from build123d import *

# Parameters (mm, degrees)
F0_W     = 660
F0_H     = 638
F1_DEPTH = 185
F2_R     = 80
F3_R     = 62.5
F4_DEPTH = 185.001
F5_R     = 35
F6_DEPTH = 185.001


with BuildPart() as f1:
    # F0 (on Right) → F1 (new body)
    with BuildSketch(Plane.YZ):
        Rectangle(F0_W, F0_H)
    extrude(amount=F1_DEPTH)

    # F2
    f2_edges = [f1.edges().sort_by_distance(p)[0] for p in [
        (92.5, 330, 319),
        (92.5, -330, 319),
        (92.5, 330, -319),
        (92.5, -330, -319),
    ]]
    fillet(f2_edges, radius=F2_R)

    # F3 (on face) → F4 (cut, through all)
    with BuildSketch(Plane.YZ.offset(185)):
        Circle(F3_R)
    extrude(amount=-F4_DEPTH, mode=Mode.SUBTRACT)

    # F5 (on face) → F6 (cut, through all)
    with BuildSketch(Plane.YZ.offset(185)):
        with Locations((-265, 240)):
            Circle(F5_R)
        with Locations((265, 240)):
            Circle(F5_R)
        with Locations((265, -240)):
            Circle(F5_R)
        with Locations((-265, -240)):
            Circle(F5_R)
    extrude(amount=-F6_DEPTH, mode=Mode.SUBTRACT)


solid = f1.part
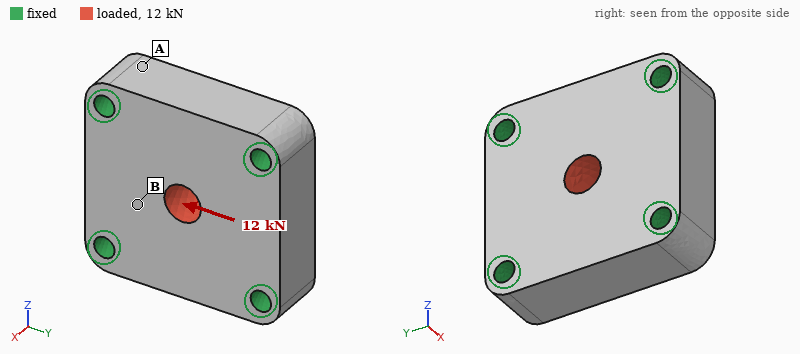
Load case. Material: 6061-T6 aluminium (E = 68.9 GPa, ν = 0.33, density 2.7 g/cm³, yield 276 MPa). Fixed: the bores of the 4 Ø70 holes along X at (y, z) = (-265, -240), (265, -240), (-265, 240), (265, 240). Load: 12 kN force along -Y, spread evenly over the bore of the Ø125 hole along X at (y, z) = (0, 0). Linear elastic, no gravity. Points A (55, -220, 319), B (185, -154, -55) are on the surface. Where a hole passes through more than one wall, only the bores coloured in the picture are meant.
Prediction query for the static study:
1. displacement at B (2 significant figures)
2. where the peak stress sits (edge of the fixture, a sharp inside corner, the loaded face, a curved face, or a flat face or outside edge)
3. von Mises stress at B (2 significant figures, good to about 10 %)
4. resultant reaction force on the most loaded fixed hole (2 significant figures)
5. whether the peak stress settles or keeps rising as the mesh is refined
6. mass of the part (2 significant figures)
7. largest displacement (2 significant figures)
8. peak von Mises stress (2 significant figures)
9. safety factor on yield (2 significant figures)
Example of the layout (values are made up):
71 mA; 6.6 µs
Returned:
0.42 µm; the loaded face; 0.096 MPa; 3.3 kN; settles; 190 kg; 0.63 µm; 0.29 MPa; 950
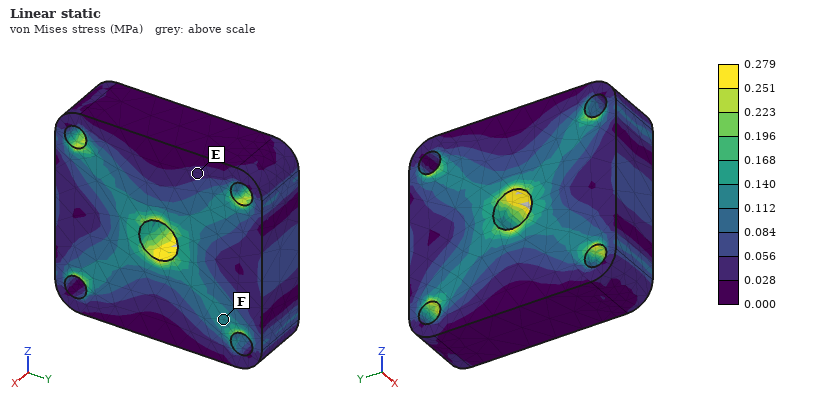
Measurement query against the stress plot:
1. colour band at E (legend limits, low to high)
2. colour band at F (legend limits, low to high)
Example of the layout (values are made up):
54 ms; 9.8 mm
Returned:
0.028 to 0.056 MPa; 0.112 to 0.140 MPa
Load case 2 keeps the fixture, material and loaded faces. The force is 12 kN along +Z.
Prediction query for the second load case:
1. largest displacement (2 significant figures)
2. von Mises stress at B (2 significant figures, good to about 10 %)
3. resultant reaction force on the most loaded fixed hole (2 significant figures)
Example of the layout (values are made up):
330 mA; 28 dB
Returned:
0.70 µm; 0.095 MPa; 3.4 kN
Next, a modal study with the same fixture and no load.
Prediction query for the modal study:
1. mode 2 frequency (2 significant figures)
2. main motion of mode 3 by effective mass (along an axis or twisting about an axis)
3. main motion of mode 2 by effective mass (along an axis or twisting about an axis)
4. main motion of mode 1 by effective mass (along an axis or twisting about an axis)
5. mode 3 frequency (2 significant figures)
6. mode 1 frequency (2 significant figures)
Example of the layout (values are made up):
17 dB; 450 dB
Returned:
2400 Hz; along Z; twisting about Y; along X; 2600 Hz; 1800 Hz
